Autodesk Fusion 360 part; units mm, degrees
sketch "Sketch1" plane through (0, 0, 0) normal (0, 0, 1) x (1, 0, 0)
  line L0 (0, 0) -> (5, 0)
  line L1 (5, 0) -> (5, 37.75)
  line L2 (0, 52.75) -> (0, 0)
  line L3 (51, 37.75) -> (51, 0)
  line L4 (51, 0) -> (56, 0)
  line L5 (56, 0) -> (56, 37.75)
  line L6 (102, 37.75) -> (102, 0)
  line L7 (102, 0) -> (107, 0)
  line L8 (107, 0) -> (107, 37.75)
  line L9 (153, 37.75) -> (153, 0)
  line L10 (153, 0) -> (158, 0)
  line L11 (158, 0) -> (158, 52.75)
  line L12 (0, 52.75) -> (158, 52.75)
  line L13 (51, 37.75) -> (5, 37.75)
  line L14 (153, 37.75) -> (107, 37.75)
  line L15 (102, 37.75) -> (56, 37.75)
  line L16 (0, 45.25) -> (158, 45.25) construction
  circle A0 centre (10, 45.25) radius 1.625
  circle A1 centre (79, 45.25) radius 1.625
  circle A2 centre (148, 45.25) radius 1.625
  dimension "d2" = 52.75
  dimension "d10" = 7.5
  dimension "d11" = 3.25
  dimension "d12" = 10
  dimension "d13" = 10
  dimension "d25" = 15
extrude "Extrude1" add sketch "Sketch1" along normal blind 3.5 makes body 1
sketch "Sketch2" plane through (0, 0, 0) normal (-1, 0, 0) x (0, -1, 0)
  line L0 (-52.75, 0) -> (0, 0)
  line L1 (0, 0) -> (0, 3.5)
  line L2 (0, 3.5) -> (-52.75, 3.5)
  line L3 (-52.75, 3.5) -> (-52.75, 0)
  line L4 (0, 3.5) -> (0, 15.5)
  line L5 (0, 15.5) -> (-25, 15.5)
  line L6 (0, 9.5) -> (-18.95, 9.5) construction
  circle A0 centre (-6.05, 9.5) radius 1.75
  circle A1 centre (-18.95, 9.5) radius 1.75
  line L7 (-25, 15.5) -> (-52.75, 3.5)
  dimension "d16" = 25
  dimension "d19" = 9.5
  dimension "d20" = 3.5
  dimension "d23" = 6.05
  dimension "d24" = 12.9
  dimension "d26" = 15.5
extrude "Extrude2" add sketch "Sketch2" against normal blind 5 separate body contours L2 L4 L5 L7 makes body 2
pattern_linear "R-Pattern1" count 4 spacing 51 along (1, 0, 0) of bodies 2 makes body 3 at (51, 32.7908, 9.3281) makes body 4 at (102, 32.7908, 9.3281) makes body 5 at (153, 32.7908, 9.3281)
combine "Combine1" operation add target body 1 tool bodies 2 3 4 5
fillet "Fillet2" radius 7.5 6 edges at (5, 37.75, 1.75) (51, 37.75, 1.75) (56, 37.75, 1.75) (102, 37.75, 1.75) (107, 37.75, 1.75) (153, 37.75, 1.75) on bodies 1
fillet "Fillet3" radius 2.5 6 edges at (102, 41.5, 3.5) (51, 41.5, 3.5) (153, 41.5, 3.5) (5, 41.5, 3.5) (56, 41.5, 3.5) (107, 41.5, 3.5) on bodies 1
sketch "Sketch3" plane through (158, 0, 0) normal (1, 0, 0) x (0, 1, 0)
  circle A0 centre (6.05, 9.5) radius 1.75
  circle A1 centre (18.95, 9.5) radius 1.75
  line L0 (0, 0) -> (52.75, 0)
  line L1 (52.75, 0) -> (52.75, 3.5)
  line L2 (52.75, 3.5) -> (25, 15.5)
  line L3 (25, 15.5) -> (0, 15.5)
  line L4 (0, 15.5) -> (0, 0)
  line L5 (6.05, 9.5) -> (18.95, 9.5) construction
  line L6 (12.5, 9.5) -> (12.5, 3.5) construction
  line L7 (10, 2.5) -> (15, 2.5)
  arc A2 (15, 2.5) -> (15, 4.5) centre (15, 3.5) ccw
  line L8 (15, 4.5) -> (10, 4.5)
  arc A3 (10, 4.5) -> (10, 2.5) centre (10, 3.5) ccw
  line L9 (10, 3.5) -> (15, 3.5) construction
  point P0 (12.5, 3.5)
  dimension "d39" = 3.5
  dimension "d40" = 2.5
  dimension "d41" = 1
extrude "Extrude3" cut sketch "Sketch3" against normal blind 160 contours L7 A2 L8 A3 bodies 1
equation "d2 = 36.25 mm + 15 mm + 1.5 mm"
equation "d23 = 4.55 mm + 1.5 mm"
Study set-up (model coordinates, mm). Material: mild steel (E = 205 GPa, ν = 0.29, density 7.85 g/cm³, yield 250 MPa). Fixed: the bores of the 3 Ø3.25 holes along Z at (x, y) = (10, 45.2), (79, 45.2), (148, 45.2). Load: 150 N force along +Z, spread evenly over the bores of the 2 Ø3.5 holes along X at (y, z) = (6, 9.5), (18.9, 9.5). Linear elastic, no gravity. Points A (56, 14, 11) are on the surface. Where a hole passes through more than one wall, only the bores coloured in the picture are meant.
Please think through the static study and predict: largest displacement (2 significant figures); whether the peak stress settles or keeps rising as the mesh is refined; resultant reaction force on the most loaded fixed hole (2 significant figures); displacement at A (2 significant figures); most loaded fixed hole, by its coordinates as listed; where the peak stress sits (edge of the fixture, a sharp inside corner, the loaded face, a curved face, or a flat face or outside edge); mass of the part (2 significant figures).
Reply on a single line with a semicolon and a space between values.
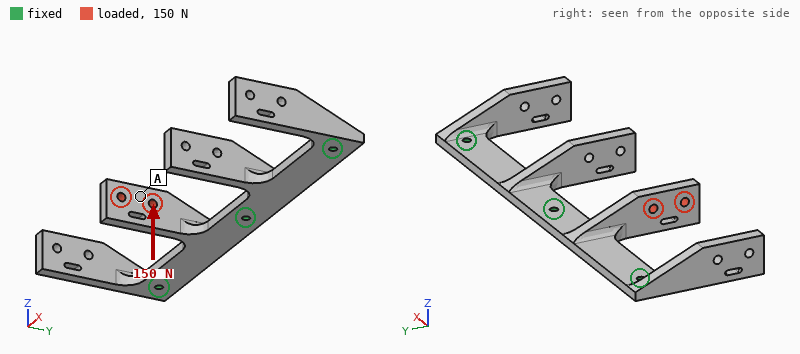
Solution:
0.24 mm; keeps rising; 110 N; 0.17 mm; (79, 45.2); edge of the fixture; 160 g
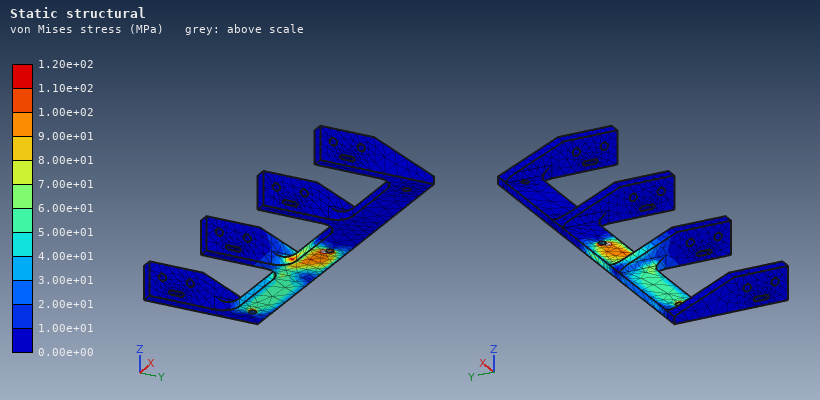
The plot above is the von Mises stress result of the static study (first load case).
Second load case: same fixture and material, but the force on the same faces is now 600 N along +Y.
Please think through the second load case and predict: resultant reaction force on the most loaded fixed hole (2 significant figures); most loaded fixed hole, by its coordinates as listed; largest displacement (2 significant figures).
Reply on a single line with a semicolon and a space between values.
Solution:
450 N; (79, 45.2); 0.22 mm
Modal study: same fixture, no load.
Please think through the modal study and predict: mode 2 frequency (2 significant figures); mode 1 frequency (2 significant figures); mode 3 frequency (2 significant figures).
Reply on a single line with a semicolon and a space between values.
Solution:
1100 Hz; 1100 Hz; 1700 Hz
